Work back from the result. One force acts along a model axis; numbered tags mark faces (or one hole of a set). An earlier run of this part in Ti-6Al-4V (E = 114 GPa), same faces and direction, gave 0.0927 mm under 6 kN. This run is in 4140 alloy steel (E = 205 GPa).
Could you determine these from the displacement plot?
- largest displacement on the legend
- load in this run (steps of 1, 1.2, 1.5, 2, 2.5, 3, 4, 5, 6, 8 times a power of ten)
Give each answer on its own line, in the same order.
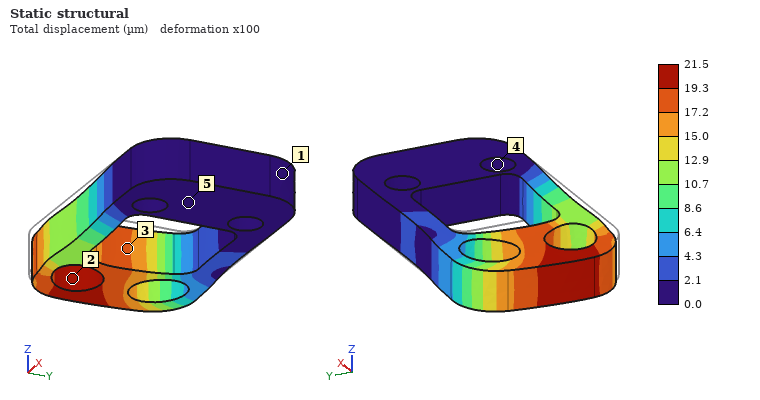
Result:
21.5 µm
2.5 kN
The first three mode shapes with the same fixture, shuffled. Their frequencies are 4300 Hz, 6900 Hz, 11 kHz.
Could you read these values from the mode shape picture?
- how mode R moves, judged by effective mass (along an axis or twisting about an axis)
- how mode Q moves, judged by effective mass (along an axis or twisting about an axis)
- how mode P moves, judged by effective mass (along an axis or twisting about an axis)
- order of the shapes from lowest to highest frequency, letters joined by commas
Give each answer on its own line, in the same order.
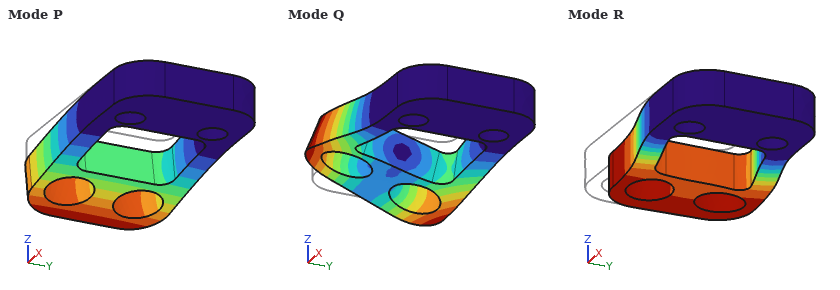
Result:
along Y
twisting about X
along Z
P, R, Q
